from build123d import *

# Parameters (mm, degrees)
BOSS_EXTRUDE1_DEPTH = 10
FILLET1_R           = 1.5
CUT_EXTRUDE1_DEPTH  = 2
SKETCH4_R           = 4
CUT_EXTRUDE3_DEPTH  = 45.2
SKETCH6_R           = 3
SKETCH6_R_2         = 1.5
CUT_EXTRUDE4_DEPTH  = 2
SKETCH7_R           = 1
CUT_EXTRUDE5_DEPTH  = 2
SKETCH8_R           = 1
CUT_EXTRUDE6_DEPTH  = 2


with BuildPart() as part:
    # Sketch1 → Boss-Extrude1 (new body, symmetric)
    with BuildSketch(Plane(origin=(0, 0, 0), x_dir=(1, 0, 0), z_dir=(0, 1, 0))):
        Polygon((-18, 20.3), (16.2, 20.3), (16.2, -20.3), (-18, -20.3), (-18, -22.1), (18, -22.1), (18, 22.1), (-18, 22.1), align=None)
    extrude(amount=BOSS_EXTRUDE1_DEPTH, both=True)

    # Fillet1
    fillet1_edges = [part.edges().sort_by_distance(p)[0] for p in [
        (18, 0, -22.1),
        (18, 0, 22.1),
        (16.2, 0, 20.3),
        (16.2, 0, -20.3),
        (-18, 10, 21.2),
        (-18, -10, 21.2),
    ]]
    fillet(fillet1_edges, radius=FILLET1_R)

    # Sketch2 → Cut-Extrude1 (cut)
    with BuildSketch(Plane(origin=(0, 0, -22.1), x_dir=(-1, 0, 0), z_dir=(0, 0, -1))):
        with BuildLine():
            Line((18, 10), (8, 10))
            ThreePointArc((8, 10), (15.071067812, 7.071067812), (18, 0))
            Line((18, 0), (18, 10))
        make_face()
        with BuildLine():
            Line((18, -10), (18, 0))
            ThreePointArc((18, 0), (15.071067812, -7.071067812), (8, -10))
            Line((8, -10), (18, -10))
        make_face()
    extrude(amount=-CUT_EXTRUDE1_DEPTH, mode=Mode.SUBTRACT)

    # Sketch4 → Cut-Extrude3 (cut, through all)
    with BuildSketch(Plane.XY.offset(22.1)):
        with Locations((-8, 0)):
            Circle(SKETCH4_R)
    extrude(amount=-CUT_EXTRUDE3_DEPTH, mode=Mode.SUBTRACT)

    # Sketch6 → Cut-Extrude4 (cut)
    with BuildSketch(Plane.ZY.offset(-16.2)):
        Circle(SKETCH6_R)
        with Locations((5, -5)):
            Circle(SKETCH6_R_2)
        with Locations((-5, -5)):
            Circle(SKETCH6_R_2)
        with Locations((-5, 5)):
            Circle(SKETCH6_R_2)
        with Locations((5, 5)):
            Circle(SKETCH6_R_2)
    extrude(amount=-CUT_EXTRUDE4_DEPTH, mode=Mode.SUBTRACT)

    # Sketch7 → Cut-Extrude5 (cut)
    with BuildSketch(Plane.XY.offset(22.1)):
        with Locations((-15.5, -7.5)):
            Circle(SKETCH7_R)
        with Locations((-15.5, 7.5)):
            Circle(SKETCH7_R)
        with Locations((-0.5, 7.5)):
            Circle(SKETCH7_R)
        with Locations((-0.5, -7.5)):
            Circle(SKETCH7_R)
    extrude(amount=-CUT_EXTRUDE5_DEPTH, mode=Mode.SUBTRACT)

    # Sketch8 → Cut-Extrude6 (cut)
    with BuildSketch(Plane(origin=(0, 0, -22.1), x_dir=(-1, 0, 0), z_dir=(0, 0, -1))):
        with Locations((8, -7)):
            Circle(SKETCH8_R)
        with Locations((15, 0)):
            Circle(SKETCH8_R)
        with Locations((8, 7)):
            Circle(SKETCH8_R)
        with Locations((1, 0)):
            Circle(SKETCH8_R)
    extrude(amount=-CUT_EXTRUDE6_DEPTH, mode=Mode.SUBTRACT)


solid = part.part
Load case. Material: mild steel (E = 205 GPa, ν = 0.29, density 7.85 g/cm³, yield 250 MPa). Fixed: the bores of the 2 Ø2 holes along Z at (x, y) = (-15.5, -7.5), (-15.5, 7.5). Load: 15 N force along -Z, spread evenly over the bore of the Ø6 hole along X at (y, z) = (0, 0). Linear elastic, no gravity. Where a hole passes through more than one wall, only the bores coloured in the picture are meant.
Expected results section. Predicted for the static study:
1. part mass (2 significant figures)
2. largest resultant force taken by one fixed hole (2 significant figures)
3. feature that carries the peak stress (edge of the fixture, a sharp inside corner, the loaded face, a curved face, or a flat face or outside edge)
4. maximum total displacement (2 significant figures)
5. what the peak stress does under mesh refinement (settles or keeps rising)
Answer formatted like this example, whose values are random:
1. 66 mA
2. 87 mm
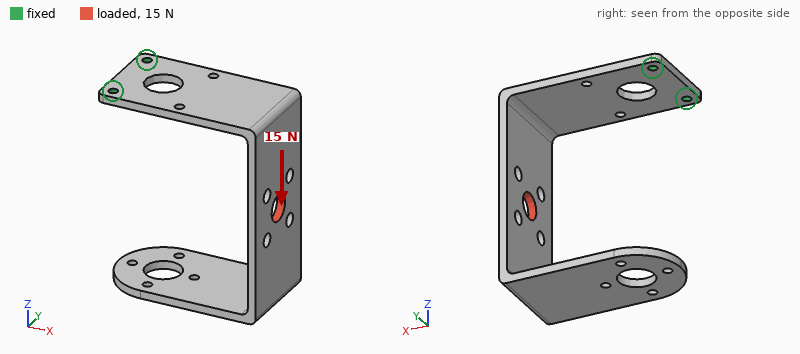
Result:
1. 29 g
2. 7.5 N
3. edge of the fixture
4. 0.25 mm
5. keeps rising
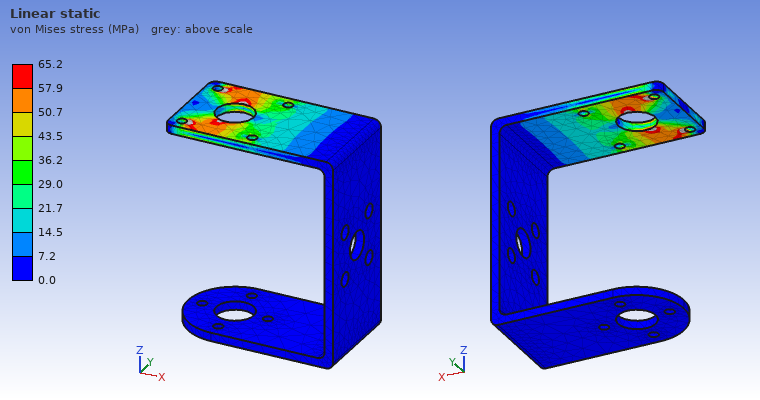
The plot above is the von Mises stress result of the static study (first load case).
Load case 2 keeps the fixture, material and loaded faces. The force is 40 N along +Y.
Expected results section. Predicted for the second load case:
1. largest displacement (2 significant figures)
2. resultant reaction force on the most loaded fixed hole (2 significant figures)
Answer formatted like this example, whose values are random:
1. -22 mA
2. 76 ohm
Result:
1. 0.37 mm
2. 97 N
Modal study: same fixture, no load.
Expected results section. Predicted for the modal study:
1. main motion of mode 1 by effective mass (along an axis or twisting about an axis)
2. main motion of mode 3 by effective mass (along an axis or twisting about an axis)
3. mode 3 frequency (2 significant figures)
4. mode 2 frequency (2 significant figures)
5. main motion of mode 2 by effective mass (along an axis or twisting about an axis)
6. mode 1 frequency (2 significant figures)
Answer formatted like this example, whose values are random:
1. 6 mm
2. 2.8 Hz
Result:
1. along X
2. along Z
3. 500 Hz
4. 320 Hz
5. along Y
6. 200 Hz
